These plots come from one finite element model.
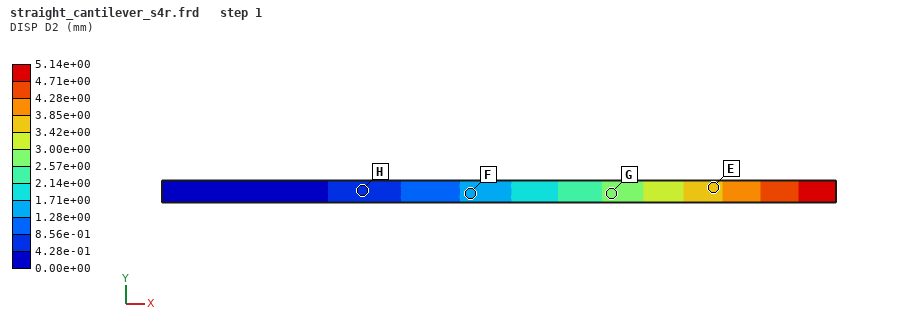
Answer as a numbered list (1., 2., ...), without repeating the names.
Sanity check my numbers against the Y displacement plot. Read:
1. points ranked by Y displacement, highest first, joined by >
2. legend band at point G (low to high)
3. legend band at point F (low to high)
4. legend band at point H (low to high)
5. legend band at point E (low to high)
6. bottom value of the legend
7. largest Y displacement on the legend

1. E > G > F > H
2. 2.57e+00 to 3.00e+00 mm
3. 1.28e+00 to 1.71e+00 mm
4. 4.28e-01 to 8.56e-01 mm
5. 3.42e+00 to 3.85e+00 mm
6. 0.00e+00 mm
7. 5.14e+00 mm
